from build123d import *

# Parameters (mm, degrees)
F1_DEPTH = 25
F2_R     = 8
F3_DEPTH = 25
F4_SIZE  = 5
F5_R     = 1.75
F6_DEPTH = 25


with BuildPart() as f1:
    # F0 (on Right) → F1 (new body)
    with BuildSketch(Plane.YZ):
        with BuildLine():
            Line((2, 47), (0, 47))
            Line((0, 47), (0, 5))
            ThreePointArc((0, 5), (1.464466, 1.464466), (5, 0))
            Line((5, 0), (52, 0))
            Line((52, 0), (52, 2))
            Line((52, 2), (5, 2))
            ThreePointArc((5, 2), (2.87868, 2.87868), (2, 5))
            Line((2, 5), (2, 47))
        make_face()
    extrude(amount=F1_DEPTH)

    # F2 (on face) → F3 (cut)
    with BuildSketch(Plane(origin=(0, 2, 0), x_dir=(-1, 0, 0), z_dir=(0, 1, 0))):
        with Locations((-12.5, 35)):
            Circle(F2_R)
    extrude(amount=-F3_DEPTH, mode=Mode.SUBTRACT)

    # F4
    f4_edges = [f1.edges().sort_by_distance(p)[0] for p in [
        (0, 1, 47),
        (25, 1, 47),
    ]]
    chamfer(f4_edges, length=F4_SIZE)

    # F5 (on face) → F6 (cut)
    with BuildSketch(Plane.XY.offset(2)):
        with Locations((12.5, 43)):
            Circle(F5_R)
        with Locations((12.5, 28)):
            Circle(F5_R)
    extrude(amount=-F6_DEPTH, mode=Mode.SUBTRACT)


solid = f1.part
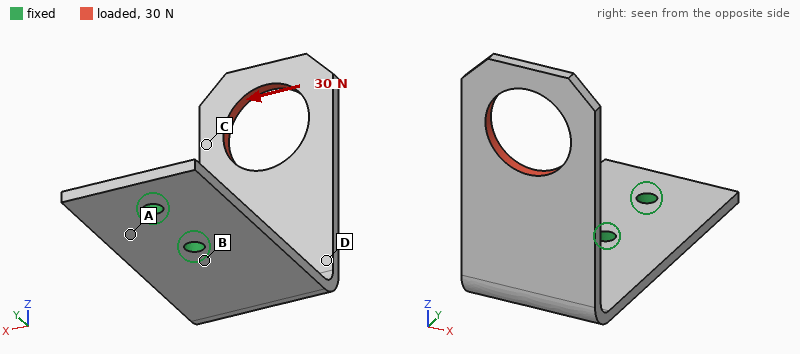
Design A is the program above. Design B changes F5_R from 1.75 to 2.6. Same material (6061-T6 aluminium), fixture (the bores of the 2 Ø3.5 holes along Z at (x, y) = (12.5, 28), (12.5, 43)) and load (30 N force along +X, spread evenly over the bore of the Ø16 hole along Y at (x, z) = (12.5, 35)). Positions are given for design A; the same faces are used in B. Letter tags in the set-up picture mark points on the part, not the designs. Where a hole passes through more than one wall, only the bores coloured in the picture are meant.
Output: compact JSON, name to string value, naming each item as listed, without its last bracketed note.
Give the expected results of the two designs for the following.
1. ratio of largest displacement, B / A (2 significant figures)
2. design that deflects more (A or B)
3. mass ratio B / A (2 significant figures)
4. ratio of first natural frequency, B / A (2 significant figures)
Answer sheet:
{"ratio of largest displacement, B / A": "0.92", "design that deflects more": "A", "mass ratio B / A": "0.99", "ratio of first natural frequency, B / A": "1.0"}
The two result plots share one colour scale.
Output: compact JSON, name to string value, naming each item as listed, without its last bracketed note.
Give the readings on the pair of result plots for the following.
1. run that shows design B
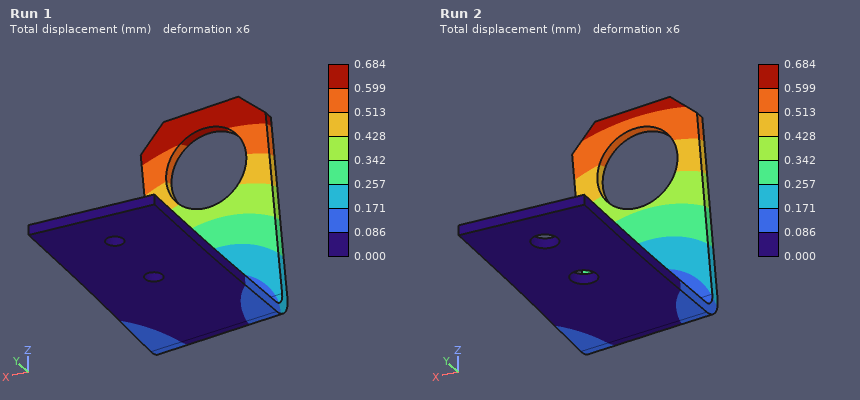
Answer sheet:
{"run that shows design B": "Run 2"}
